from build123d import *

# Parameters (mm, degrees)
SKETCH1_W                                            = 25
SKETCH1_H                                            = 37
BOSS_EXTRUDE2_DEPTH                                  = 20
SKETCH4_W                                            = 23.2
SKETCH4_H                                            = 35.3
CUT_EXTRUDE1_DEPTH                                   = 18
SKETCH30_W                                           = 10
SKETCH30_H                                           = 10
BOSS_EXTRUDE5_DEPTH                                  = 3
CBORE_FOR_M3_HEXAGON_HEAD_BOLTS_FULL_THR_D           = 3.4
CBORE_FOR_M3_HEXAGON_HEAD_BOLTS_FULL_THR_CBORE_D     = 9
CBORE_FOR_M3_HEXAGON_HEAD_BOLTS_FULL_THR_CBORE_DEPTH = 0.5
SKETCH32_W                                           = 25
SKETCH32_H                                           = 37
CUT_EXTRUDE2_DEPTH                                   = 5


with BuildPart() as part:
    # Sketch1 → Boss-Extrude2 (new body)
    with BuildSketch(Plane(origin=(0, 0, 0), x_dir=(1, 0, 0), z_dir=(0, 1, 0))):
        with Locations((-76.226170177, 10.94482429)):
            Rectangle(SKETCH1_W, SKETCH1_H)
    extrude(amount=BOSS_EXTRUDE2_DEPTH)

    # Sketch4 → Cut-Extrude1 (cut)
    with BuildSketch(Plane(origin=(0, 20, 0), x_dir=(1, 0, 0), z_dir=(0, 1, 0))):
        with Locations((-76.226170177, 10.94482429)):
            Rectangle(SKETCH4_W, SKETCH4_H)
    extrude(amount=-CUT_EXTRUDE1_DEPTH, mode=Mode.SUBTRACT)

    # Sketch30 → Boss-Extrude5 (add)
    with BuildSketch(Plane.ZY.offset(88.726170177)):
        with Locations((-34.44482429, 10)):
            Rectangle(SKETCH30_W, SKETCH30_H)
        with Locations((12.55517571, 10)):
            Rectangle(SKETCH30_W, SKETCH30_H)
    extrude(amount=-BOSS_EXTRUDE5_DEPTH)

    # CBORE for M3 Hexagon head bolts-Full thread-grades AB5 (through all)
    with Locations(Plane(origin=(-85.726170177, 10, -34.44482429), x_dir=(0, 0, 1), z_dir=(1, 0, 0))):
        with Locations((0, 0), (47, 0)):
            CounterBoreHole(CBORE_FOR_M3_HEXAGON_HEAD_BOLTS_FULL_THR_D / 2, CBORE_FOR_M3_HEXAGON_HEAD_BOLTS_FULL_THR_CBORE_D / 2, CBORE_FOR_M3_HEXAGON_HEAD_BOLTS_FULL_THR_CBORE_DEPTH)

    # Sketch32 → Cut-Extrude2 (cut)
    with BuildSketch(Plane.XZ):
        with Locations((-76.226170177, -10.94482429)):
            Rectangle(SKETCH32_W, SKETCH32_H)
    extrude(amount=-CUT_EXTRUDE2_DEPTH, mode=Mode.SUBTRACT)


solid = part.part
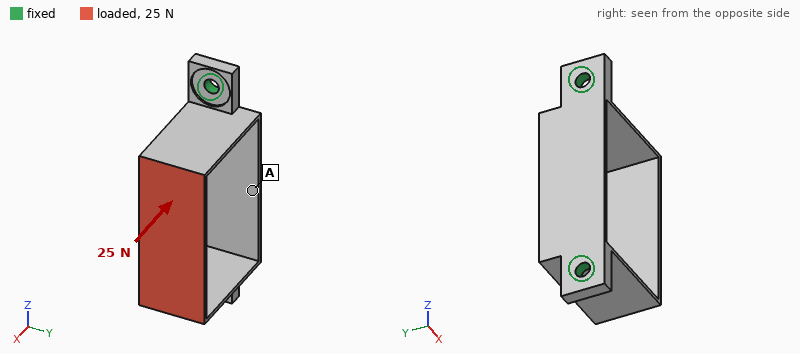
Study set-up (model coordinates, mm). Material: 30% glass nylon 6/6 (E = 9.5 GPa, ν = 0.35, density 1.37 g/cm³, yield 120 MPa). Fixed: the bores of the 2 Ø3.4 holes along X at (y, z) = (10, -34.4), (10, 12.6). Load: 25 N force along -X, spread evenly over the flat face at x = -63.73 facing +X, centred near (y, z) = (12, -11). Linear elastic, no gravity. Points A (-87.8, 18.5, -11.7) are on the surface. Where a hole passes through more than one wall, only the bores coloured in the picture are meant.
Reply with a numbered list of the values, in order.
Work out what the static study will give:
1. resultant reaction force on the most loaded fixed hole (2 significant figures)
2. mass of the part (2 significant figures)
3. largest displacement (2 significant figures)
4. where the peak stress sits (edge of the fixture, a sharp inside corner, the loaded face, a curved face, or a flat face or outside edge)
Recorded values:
1. 13 N
2. 2.9 g
3. 0.69 mm
4. a flat face or outside edge
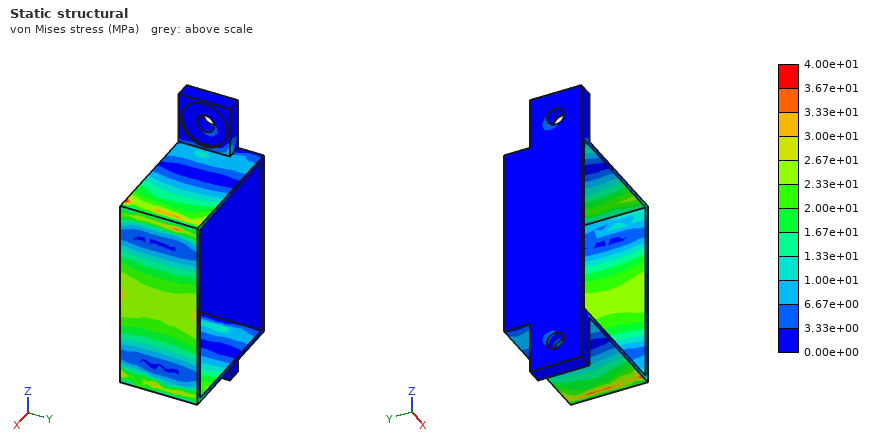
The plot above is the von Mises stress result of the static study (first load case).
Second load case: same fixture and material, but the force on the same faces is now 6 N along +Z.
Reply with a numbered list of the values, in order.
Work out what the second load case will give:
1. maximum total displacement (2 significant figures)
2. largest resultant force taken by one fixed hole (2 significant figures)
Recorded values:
1. 0.54 mm
2. 3.5 N
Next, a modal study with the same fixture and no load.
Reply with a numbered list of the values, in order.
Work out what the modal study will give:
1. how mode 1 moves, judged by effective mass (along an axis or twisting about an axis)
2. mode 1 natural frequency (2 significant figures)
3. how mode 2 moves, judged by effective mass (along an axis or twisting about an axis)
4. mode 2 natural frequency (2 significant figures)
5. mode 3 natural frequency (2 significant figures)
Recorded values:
1. along Z
2. 560 Hz
3. along X
4. 1300 Hz
5. 1700 Hz
